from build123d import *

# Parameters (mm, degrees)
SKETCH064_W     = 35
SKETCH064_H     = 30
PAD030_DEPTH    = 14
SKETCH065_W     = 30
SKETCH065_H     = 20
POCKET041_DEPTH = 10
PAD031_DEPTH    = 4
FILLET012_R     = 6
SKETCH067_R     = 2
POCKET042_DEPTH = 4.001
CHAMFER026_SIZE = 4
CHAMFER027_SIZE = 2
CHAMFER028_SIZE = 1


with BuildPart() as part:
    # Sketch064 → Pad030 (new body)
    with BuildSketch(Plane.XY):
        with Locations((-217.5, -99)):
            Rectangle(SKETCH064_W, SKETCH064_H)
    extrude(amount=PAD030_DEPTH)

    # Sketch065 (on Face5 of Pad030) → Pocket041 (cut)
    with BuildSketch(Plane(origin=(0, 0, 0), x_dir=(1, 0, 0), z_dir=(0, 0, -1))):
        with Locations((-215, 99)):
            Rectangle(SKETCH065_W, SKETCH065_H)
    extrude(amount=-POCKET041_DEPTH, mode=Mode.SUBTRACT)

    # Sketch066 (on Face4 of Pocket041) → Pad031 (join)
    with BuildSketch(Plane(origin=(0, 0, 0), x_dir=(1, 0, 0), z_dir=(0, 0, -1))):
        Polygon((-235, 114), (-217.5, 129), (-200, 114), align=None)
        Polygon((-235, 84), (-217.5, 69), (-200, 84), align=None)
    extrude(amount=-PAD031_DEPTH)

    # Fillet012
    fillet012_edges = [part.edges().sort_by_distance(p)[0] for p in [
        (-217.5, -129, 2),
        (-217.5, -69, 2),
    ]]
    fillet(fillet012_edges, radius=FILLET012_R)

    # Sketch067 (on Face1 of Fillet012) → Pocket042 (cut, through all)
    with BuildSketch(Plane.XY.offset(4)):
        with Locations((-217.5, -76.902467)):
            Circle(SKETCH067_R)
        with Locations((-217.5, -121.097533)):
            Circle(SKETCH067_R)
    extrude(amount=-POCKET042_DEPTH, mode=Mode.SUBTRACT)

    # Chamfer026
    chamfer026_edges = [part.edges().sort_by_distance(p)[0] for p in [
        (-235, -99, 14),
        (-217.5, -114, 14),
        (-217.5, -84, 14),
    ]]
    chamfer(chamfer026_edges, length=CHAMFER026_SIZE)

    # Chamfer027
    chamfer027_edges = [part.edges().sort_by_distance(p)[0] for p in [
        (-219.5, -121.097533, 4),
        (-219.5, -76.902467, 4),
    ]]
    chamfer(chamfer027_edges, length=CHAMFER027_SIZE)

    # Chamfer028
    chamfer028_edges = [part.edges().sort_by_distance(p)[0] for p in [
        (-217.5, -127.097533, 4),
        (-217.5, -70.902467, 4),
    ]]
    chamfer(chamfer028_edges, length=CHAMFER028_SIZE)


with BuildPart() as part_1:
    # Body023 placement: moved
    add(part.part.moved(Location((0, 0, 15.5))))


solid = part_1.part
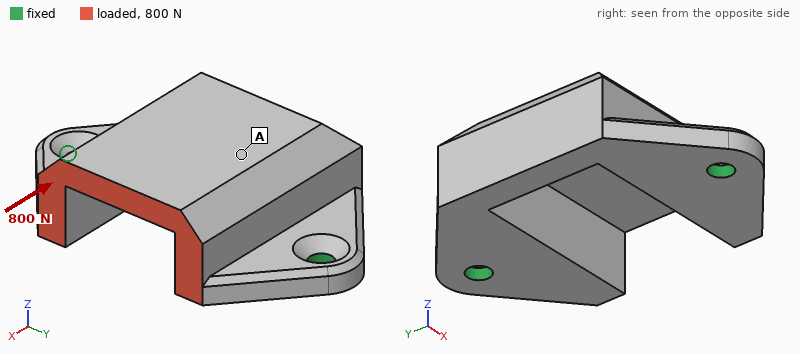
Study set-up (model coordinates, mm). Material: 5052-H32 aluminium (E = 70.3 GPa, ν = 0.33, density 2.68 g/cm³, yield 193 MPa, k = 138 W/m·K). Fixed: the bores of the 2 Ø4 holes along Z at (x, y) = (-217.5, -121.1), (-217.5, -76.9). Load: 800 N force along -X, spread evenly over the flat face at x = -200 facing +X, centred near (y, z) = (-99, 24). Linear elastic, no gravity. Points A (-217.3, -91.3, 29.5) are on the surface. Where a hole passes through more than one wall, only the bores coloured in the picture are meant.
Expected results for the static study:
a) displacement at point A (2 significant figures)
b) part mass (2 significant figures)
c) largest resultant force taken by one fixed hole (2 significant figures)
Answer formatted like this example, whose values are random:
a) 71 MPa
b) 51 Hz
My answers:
a) 49 µm
b) 26 g
c) 430 N
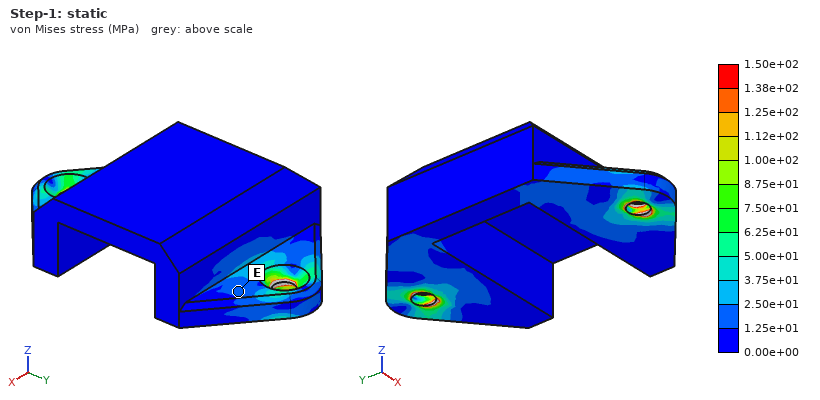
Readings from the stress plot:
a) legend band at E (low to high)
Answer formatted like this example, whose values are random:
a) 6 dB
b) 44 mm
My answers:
a) 1.25e+01 to 2.50e+01 MPa
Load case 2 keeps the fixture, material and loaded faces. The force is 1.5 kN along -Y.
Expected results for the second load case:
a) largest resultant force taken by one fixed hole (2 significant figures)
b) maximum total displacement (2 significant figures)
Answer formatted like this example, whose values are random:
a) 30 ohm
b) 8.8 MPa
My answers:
a) 940 N
b) 43 µm
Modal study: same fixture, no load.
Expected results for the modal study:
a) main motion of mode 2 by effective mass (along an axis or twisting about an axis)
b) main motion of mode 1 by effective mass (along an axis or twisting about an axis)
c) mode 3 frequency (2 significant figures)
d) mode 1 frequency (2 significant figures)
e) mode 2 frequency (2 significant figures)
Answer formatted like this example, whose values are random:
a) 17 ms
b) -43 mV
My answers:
a) along Z
b) along X
c) 11 kHz
d) 3300 Hz
e) 9800 Hz
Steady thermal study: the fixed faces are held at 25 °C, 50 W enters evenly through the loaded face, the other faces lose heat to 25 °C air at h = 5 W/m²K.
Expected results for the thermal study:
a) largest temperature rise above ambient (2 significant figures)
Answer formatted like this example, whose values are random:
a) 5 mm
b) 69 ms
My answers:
a) 55 K
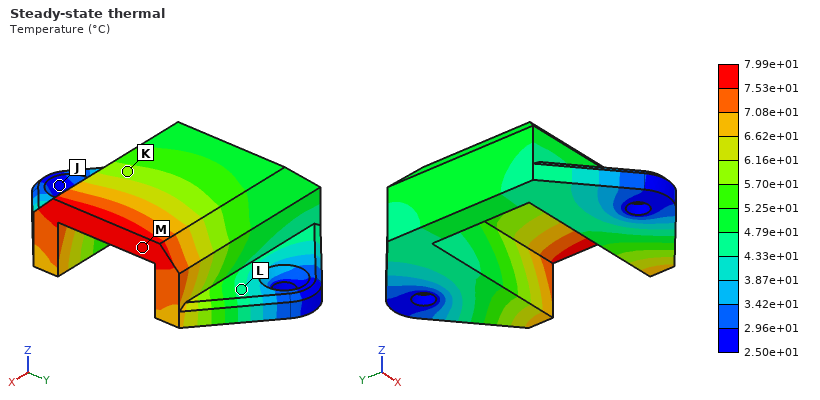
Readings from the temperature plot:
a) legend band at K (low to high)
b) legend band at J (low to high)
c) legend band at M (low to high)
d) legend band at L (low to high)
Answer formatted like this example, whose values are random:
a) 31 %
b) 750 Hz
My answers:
a) 5.70e+01 to 6.16e+01 °C
b) 2.50e+01 to 2.96e+01 °C
c) 7.53e+01 to 7.99e+01 °C
d) 4.33e+01 to 4.79e+01 °C
